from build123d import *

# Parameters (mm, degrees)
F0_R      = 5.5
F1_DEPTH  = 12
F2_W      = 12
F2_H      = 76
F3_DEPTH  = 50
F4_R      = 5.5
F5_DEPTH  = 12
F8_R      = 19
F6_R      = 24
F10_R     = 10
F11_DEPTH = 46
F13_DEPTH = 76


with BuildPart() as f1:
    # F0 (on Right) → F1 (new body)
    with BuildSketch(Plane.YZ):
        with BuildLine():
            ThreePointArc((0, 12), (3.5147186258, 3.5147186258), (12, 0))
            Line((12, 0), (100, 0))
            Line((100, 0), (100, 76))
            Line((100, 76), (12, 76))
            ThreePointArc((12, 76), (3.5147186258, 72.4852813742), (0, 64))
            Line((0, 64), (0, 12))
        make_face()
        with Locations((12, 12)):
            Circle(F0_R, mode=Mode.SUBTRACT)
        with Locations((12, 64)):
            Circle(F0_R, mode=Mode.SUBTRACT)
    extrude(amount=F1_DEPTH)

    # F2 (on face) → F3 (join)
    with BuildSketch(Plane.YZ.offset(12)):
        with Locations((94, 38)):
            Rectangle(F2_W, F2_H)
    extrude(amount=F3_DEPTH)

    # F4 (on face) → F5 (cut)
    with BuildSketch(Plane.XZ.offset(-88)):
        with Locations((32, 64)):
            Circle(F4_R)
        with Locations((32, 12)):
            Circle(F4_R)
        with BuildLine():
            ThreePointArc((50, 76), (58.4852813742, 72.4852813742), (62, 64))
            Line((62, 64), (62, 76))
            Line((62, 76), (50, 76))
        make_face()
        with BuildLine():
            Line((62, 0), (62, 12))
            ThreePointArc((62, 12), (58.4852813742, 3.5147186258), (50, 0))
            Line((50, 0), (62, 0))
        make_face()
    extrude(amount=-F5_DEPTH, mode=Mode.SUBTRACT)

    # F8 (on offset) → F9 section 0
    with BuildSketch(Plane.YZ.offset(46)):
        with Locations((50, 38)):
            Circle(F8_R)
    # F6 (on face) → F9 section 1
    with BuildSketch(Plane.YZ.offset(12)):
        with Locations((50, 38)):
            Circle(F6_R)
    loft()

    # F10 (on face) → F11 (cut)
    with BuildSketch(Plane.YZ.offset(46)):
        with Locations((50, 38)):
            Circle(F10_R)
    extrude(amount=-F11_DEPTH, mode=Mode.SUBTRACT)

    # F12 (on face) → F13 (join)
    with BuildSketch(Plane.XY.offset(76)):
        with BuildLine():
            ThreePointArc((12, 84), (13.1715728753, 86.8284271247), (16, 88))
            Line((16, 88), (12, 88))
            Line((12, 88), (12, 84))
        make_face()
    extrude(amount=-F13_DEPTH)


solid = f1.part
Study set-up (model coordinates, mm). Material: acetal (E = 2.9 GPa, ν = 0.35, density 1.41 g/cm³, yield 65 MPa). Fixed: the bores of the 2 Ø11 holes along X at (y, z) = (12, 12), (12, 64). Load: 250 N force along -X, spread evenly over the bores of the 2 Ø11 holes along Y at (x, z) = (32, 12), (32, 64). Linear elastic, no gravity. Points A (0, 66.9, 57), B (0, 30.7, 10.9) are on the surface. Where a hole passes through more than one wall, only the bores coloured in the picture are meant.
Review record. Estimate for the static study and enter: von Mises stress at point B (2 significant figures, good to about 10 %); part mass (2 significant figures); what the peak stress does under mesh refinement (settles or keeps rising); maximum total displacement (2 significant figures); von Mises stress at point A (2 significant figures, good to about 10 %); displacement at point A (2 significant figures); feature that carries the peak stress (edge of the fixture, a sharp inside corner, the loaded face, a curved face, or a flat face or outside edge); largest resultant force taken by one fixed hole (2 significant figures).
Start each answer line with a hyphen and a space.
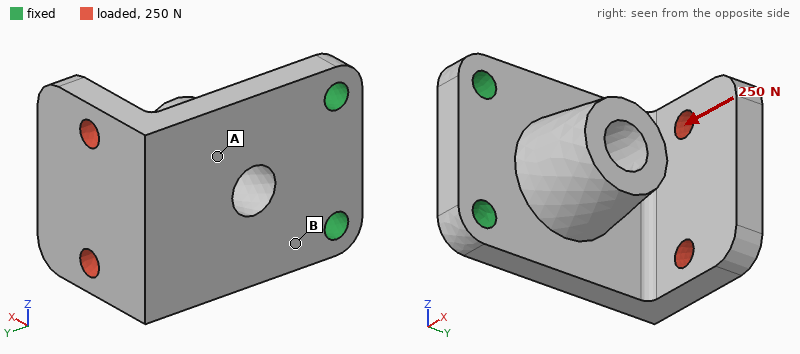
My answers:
- 7.7 MPa
- 230 g
- keeps rising
- 1.5 mm
- 2.8 MPa
- 0.59 mm
- edge of the fixture
- 130 N
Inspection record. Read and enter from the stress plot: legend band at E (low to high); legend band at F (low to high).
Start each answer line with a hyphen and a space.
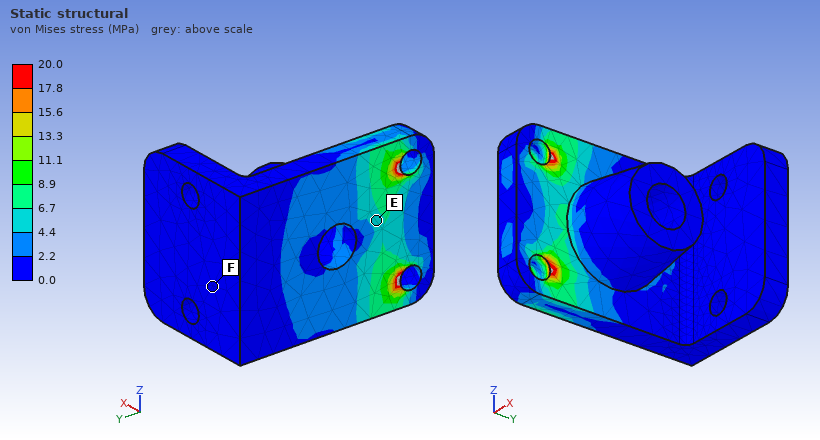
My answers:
- 4.4 to 6.7 MPa
- 0.0 to 2.2 MPa
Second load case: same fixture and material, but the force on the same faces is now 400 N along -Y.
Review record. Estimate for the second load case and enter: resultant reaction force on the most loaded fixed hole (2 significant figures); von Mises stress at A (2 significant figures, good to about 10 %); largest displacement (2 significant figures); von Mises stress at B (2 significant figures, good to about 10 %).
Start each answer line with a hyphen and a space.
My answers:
- 210 N
- 3.7 MPa
- 1.4 mm
- 4.2 MPa
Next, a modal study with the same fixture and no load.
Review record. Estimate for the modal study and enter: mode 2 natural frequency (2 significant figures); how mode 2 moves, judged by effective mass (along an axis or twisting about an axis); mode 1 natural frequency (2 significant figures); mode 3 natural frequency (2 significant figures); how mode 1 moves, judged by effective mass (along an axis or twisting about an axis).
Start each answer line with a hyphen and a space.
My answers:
- 540 Hz
- along Z
- 220 Hz
- 660 Hz
- along X
